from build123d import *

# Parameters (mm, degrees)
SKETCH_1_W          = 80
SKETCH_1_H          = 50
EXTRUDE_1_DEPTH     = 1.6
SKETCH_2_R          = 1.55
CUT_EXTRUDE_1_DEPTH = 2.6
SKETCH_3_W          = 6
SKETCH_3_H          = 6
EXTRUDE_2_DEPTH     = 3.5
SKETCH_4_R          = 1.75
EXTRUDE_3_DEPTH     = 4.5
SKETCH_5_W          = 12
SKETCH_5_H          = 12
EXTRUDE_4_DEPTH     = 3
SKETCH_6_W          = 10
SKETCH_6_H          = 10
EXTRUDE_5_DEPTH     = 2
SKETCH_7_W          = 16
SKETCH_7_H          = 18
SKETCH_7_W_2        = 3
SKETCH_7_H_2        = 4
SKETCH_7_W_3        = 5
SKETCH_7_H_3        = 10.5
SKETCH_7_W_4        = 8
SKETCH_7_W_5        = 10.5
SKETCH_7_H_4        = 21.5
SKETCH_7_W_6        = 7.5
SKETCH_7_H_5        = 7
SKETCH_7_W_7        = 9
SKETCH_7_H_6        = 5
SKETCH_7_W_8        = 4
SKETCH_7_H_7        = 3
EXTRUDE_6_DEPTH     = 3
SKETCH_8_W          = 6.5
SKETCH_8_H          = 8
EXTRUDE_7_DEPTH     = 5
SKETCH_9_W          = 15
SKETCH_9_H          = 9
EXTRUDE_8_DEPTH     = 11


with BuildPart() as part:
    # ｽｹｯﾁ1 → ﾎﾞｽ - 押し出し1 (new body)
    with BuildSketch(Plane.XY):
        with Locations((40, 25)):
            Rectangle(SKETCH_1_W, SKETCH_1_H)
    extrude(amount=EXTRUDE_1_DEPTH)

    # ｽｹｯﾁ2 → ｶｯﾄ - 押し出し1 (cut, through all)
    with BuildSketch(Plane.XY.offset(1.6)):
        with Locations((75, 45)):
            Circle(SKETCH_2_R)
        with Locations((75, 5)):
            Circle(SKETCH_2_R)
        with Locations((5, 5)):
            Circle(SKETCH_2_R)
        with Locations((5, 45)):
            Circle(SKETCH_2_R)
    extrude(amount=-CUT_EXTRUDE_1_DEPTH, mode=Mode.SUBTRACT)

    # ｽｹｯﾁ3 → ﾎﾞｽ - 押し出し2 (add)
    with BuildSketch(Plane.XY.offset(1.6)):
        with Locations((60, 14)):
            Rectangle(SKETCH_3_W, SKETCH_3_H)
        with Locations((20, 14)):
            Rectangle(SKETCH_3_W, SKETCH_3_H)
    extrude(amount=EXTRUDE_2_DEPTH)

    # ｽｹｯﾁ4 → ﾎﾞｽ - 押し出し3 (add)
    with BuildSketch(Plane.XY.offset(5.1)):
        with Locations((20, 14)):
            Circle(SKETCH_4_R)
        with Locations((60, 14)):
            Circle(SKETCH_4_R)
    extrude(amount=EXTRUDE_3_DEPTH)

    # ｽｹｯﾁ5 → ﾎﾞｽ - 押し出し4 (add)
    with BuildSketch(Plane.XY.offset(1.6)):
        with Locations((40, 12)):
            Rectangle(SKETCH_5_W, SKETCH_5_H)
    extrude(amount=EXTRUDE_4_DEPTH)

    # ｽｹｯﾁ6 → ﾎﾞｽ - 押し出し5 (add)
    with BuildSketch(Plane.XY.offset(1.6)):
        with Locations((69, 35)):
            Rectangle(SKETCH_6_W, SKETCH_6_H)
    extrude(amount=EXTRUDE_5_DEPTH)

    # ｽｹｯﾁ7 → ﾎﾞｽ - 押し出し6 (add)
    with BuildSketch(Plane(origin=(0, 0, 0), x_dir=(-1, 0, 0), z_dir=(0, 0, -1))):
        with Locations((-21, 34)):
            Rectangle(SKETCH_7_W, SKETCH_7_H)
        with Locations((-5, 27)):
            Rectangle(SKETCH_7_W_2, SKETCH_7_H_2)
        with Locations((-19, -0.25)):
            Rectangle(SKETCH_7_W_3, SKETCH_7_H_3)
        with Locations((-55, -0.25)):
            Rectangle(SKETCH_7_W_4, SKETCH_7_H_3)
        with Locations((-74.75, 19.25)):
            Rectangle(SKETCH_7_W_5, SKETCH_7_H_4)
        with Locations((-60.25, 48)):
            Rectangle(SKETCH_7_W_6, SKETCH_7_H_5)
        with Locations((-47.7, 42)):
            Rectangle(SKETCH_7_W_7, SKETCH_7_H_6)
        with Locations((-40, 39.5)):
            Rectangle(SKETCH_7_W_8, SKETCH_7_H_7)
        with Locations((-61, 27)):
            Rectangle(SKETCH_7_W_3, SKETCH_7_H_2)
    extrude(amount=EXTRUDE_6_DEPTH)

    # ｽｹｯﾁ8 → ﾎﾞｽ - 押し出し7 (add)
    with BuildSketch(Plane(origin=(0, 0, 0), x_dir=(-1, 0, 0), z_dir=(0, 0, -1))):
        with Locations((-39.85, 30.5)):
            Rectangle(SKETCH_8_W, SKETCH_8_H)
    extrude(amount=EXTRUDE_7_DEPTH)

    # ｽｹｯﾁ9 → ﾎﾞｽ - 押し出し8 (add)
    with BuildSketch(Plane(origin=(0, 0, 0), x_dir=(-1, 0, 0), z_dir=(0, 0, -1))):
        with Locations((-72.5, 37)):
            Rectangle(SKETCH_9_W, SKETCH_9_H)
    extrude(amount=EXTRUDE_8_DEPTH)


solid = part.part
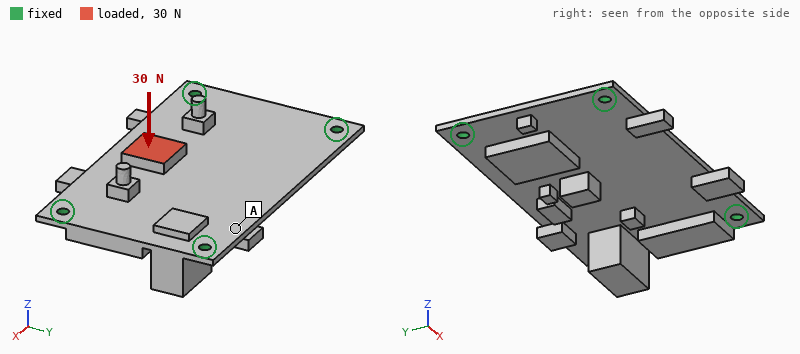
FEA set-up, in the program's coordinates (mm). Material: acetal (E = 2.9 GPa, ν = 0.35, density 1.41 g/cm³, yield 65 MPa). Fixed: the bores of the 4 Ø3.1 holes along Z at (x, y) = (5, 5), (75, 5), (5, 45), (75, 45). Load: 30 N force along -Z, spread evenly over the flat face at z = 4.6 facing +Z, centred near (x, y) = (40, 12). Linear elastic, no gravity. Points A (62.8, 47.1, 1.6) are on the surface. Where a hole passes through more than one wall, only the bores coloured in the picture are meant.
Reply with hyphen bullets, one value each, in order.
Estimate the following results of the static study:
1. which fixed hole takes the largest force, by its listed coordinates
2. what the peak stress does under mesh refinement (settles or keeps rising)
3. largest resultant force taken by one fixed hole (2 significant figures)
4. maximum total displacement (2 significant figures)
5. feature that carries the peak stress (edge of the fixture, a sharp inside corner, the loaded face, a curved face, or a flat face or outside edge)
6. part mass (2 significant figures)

- (75, 5)
- keeps rising
- 16 N
- 1.1 mm
- edge of the fixture
- 16 g
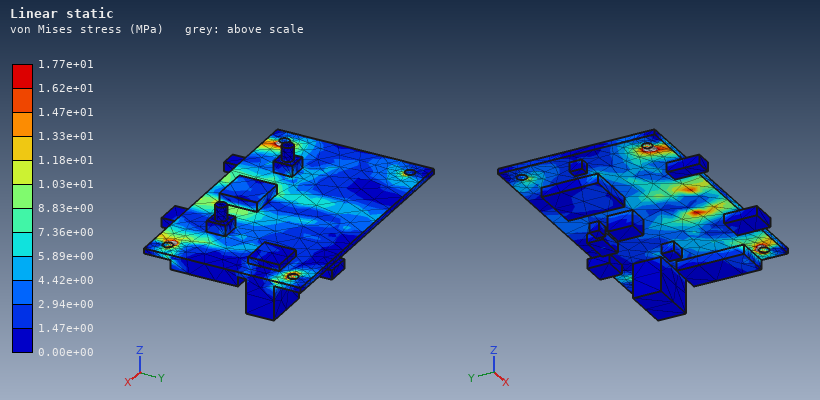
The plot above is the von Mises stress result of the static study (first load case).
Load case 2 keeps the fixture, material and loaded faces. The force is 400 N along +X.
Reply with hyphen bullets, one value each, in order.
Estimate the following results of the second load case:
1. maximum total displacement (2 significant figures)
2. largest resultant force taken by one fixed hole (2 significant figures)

- 0.91 mm
- 130 N
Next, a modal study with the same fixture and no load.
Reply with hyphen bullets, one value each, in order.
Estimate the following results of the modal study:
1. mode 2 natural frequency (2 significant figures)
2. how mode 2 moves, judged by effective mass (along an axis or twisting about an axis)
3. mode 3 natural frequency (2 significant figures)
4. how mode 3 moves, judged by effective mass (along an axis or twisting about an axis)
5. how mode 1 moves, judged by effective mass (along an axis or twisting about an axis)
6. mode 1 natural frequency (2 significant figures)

- 740 Hz
- twisting about X
- 1100 Hz
- twisting about Y
- along Z
- 430 Hz
